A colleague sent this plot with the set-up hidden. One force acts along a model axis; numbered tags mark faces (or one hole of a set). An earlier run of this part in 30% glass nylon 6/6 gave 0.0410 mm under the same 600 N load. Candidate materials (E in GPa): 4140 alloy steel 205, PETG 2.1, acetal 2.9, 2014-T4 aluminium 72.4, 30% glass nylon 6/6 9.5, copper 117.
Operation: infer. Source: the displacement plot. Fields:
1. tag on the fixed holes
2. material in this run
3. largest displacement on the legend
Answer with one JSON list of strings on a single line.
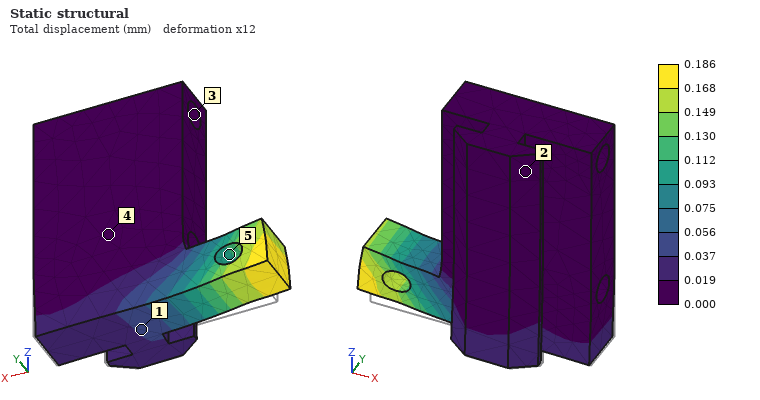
["3", "PETG", "0.186 mm"]
